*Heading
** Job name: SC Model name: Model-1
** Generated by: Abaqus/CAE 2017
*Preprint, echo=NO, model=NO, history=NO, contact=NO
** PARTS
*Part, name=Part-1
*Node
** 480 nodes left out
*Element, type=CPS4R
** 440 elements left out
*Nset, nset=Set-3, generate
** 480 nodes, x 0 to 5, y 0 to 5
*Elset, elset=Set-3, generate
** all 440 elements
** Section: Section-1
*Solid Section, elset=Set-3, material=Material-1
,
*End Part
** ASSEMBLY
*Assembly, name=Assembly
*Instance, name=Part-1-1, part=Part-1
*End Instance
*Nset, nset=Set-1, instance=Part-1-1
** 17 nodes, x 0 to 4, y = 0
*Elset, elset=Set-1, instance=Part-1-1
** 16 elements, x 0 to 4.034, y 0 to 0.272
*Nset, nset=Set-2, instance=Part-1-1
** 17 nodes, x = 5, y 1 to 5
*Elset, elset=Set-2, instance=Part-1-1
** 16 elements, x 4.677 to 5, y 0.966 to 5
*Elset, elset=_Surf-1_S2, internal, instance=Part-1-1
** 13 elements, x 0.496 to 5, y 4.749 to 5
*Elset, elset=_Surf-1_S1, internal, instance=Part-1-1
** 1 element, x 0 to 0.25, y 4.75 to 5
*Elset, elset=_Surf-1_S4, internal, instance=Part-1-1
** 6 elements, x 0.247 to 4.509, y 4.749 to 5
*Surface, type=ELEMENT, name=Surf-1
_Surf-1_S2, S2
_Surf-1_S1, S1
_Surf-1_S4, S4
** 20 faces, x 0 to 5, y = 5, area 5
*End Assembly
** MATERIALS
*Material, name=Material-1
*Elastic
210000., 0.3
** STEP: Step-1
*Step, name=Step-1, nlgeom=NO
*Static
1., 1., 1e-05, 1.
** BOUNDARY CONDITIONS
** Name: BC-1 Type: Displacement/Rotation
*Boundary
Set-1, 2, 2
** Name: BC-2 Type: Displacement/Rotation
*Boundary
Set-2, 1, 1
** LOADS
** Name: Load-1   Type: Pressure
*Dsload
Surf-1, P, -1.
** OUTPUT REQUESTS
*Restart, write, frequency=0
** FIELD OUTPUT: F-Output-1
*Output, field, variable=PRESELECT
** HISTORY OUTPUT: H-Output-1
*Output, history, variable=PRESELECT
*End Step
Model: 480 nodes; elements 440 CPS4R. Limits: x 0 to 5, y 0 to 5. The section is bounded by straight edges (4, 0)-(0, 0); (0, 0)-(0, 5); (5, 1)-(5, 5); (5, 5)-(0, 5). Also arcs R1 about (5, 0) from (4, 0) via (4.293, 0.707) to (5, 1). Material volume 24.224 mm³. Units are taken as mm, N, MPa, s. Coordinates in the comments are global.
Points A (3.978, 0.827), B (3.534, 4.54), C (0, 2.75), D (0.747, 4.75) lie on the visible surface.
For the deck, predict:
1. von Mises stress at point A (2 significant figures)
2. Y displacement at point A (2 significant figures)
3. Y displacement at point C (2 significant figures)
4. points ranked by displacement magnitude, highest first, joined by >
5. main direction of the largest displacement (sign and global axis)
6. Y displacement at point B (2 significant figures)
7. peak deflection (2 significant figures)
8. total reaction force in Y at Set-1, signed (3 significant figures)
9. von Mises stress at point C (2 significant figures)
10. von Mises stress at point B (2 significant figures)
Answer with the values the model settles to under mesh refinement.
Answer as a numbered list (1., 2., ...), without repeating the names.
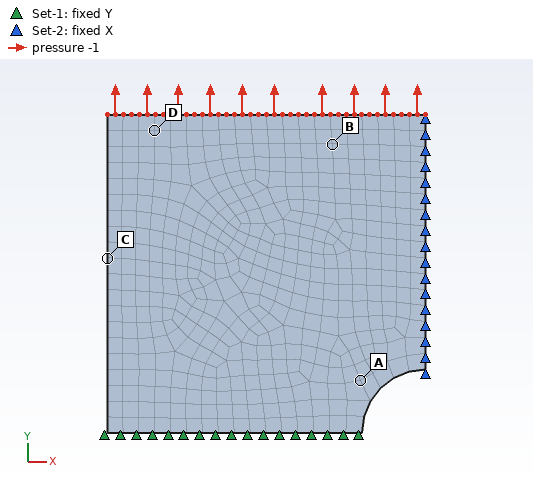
1. 1.5 MPa
2. 8.3e-06 mm
3. 1.2e-05 mm
4. B > D > C > A
5. +Y
6. 2.6e-05 mm
7. 2.9e-05 mm
8. -5.00 N
9. 0.99 MPa
10. 0.95 MPa
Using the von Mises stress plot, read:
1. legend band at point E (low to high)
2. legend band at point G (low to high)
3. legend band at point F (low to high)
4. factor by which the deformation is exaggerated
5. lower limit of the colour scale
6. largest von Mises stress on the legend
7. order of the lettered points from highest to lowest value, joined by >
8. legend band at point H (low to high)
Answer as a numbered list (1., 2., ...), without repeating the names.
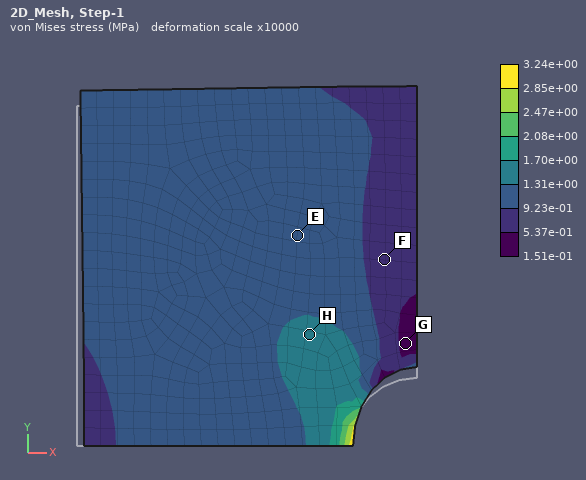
1. 9.23e-01 to 1.31e+00 MPa
2. 1.51e-01 to 5.37e-01 MPa
3. 5.37e-01 to 9.23e-01 MPa
4. 10000
5. 1.51e-01 MPa
6. 3.24e+00 MPa
7. H > E > F > G
8. 1.31e+00 to 1.70e+00 MPa
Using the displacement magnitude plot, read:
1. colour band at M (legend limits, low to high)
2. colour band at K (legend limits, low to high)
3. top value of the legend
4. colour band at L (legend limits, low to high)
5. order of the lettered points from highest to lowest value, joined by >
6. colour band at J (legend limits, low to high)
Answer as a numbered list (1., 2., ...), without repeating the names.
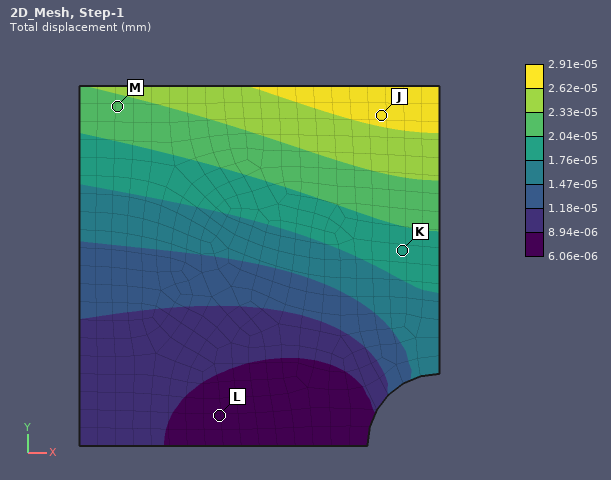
1. 2.04e-05 to 2.33e-05 mm
2. 1.76e-05 to 2.04e-05 mm
3. 2.91e-05 mm
4. 6.06e-06 to 8.94e-06 mm
5. J > M > K > L
6. 2.62e-05 to 2.91e-05 mm
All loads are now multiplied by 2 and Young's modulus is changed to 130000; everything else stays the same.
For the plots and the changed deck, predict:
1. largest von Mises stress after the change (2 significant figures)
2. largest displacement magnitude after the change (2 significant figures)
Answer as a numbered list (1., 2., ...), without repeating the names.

1. 6.5 MPa
2. 9.4e-05 mm
